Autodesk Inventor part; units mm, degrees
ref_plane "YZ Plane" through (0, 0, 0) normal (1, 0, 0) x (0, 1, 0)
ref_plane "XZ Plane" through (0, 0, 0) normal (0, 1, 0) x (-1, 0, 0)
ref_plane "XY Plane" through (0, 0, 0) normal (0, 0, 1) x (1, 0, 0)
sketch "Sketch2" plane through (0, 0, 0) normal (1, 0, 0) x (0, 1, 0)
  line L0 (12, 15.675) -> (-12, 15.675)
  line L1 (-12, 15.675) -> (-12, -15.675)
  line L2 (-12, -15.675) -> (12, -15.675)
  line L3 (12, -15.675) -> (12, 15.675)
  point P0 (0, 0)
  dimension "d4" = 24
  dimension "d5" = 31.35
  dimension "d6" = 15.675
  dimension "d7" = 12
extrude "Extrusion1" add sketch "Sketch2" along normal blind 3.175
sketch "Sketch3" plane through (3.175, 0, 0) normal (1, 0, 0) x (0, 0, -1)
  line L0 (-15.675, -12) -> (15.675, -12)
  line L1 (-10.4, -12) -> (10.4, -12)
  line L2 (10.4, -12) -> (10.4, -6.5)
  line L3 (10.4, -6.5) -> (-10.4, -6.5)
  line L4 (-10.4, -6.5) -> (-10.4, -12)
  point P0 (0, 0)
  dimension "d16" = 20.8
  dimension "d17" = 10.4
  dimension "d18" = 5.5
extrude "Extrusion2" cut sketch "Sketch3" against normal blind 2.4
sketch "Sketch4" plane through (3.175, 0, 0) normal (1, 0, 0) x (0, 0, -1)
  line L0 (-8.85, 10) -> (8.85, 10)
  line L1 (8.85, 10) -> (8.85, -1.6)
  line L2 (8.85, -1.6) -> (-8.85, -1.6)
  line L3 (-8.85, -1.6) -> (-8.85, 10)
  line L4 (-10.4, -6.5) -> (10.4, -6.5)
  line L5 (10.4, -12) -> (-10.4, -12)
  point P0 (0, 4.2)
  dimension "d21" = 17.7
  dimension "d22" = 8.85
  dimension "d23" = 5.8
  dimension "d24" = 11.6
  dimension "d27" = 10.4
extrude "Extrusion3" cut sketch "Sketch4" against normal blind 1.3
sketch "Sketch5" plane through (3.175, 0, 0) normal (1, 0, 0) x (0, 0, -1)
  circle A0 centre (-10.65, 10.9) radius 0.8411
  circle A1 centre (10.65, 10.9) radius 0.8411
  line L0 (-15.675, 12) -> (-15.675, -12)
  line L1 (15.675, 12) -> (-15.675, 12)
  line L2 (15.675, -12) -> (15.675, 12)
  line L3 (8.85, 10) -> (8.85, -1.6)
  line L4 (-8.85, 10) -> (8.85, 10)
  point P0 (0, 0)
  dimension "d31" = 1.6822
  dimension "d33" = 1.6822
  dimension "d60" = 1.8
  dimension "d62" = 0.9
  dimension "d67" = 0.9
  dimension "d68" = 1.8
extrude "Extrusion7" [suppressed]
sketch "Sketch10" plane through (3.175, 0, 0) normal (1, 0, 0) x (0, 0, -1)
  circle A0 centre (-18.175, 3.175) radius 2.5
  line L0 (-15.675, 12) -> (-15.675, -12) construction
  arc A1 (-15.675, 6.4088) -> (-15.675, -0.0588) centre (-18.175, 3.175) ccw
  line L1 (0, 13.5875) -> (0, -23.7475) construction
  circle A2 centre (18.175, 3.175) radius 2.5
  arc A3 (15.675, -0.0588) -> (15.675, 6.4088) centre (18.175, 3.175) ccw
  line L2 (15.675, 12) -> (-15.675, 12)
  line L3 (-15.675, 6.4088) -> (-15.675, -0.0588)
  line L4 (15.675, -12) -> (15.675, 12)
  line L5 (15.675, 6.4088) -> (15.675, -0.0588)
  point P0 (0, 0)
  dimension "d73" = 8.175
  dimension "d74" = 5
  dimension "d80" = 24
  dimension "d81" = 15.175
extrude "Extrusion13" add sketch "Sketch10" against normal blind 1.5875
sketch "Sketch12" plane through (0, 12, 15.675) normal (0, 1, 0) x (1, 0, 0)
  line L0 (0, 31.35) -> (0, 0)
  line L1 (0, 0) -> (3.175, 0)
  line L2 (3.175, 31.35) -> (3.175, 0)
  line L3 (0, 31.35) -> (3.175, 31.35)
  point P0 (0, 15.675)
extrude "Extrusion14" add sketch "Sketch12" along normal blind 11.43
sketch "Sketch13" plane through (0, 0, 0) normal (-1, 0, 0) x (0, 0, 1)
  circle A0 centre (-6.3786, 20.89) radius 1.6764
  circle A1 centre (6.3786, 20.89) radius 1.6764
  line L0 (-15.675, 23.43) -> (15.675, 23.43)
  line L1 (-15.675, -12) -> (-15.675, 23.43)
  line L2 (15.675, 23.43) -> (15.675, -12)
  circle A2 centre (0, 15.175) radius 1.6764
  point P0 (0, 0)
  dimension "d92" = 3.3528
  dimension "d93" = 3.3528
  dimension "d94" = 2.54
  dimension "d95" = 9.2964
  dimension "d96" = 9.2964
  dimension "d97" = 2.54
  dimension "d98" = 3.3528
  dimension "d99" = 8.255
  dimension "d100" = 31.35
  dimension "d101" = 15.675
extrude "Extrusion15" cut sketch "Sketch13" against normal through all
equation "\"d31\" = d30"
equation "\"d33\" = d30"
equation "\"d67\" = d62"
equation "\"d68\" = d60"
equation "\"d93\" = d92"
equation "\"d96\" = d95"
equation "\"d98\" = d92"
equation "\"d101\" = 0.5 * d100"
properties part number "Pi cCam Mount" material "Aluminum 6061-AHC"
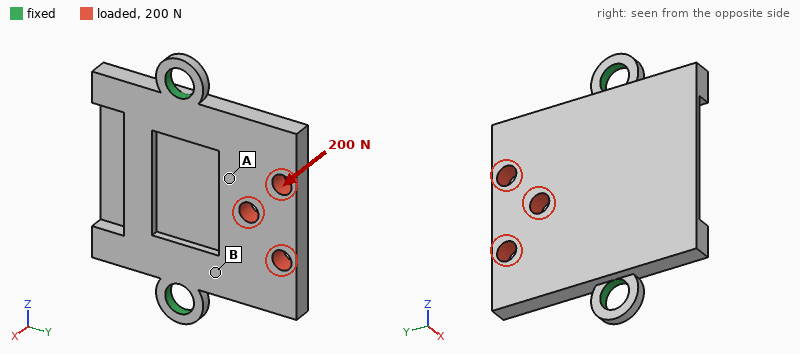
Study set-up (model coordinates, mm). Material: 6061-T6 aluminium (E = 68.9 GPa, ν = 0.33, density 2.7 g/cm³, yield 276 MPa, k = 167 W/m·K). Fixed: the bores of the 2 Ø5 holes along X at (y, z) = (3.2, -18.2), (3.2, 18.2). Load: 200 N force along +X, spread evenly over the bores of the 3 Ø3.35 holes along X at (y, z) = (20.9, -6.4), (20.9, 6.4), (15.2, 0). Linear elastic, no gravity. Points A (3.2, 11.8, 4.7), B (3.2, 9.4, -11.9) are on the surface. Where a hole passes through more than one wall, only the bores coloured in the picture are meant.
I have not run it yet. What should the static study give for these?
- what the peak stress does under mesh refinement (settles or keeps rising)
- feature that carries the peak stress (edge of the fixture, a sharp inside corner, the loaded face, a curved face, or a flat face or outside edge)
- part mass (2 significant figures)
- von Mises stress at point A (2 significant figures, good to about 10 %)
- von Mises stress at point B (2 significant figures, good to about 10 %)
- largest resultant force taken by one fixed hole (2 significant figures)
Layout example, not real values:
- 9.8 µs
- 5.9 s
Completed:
- keeps rising
- edge of the fixture
- 8.1 g
- 31 MPa
- 67 MPa
- 240 N
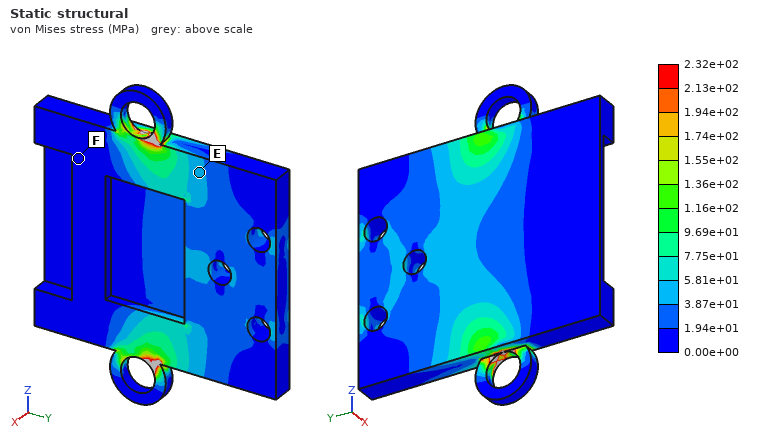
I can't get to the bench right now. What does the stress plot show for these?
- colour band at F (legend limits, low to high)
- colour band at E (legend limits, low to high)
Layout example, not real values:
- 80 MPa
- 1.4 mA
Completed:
- 0.00e+00 to 1.94e+01 MPa
- 3.87e+01 to 5.81e+01 MPa
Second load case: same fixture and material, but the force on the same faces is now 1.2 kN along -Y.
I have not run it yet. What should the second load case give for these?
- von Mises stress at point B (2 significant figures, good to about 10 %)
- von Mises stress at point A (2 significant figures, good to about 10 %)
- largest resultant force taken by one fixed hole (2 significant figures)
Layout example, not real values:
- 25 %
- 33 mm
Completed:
- 30 MPa
- 12 MPa
- 610 N
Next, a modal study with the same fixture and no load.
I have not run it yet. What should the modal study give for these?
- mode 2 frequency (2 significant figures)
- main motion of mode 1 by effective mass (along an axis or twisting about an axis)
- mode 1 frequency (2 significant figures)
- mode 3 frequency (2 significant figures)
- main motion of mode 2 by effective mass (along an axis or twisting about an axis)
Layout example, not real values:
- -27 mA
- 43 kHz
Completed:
- 7400 Hz
- along X
- 3400 Hz
- 8900 Hz
- along X
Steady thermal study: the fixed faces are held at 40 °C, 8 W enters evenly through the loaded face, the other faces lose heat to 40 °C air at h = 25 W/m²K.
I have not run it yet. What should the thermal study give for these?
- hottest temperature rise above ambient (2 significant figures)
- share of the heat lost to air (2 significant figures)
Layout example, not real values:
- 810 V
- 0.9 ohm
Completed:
- 15 K
- 6.1 %
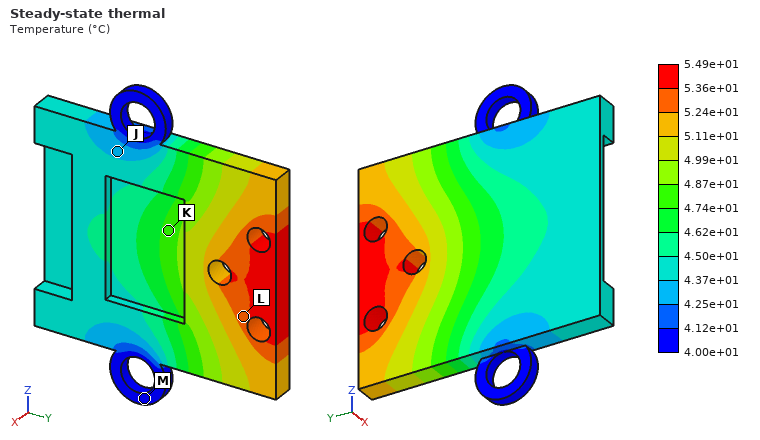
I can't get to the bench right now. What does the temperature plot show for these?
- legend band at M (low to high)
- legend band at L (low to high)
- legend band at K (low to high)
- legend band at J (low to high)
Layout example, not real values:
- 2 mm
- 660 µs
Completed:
- 4.00e+01 to 4.12e+01 °C
- 5.24e+01 to 5.36e+01 °C
- 4.74e+01 to 4.87e+01 °C
- 4.25e+01 to 4.37e+01 °C
